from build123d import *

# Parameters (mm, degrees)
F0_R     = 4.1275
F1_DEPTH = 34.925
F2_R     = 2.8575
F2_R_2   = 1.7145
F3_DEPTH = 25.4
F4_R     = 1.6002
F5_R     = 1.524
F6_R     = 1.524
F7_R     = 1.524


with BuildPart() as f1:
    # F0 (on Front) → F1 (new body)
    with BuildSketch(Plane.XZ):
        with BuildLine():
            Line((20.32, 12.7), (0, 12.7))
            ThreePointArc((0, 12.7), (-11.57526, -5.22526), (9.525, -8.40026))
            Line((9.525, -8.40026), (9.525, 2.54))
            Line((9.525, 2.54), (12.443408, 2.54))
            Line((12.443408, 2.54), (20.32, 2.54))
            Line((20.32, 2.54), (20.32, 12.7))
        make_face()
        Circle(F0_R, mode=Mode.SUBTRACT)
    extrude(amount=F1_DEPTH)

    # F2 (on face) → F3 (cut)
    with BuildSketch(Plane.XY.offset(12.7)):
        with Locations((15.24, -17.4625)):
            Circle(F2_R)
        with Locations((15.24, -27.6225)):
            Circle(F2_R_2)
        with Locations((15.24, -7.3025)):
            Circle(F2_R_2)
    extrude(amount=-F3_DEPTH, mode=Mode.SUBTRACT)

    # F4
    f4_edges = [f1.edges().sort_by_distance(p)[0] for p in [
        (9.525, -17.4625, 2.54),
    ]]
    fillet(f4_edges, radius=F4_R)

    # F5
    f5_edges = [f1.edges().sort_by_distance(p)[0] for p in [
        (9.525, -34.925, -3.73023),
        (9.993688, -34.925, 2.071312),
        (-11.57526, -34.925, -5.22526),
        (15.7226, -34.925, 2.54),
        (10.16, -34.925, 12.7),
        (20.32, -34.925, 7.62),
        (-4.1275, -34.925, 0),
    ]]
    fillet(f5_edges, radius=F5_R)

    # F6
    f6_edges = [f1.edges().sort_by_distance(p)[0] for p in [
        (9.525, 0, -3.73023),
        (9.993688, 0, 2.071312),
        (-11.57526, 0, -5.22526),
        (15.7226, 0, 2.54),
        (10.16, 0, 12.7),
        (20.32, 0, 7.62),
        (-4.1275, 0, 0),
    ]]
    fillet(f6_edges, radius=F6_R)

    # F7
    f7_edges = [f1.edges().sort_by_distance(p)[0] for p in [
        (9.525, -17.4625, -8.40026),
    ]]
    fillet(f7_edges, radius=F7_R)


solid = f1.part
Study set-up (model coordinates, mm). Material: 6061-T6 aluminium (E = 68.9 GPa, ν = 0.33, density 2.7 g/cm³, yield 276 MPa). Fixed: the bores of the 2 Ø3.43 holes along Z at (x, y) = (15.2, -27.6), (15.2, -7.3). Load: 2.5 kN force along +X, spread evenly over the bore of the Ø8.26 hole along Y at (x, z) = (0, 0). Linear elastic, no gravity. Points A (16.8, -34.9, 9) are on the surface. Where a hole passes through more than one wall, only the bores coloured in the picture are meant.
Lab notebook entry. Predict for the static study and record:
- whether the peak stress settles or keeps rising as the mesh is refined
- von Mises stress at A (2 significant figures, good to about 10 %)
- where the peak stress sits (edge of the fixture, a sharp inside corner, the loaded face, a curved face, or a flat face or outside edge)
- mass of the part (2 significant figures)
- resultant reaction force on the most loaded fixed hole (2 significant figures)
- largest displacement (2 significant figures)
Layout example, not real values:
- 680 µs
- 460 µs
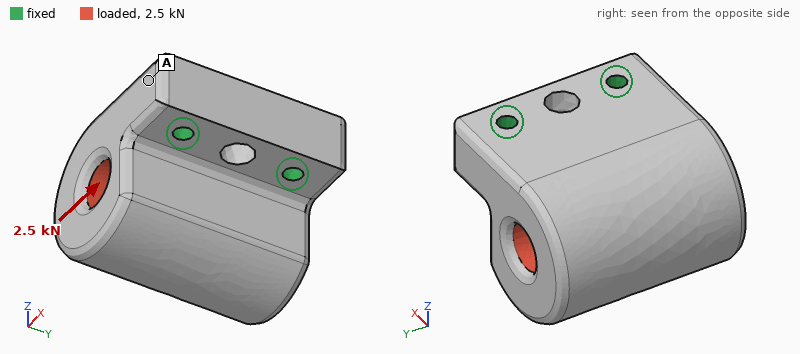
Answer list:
- keeps rising
- 11 MPa
- edge of the fixture
- 49 g
- 1.3 kN
- 32 µm
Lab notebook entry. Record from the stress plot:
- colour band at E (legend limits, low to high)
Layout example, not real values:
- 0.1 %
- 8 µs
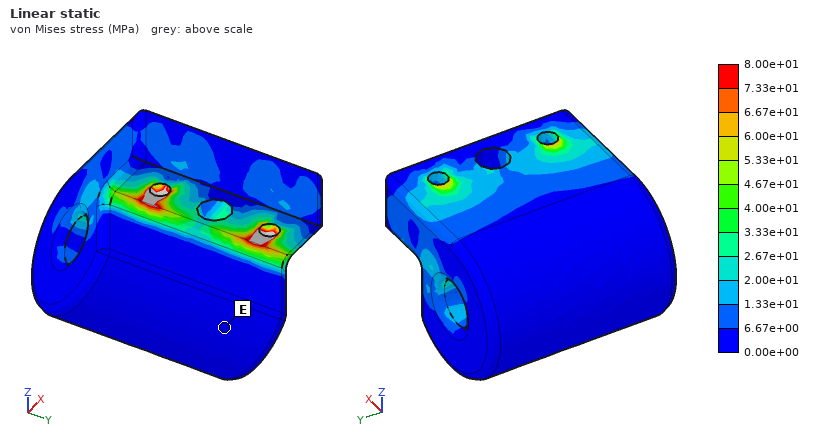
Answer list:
- 0.00e+00 to 6.67e+00 MPa
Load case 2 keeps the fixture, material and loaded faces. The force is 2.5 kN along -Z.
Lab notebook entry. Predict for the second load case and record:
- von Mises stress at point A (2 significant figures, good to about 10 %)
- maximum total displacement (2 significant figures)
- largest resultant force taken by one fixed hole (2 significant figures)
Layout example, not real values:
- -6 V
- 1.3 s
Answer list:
- 16 MPa
- 50 µm
- 1.3 kN
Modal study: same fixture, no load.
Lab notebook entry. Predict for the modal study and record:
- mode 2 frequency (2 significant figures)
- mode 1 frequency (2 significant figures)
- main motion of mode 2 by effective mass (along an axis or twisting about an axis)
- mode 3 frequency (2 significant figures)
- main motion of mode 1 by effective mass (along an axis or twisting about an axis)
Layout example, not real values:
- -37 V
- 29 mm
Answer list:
- 12 kHz
- 5800 Hz
- along Y
- 16 kHz
- along Z
